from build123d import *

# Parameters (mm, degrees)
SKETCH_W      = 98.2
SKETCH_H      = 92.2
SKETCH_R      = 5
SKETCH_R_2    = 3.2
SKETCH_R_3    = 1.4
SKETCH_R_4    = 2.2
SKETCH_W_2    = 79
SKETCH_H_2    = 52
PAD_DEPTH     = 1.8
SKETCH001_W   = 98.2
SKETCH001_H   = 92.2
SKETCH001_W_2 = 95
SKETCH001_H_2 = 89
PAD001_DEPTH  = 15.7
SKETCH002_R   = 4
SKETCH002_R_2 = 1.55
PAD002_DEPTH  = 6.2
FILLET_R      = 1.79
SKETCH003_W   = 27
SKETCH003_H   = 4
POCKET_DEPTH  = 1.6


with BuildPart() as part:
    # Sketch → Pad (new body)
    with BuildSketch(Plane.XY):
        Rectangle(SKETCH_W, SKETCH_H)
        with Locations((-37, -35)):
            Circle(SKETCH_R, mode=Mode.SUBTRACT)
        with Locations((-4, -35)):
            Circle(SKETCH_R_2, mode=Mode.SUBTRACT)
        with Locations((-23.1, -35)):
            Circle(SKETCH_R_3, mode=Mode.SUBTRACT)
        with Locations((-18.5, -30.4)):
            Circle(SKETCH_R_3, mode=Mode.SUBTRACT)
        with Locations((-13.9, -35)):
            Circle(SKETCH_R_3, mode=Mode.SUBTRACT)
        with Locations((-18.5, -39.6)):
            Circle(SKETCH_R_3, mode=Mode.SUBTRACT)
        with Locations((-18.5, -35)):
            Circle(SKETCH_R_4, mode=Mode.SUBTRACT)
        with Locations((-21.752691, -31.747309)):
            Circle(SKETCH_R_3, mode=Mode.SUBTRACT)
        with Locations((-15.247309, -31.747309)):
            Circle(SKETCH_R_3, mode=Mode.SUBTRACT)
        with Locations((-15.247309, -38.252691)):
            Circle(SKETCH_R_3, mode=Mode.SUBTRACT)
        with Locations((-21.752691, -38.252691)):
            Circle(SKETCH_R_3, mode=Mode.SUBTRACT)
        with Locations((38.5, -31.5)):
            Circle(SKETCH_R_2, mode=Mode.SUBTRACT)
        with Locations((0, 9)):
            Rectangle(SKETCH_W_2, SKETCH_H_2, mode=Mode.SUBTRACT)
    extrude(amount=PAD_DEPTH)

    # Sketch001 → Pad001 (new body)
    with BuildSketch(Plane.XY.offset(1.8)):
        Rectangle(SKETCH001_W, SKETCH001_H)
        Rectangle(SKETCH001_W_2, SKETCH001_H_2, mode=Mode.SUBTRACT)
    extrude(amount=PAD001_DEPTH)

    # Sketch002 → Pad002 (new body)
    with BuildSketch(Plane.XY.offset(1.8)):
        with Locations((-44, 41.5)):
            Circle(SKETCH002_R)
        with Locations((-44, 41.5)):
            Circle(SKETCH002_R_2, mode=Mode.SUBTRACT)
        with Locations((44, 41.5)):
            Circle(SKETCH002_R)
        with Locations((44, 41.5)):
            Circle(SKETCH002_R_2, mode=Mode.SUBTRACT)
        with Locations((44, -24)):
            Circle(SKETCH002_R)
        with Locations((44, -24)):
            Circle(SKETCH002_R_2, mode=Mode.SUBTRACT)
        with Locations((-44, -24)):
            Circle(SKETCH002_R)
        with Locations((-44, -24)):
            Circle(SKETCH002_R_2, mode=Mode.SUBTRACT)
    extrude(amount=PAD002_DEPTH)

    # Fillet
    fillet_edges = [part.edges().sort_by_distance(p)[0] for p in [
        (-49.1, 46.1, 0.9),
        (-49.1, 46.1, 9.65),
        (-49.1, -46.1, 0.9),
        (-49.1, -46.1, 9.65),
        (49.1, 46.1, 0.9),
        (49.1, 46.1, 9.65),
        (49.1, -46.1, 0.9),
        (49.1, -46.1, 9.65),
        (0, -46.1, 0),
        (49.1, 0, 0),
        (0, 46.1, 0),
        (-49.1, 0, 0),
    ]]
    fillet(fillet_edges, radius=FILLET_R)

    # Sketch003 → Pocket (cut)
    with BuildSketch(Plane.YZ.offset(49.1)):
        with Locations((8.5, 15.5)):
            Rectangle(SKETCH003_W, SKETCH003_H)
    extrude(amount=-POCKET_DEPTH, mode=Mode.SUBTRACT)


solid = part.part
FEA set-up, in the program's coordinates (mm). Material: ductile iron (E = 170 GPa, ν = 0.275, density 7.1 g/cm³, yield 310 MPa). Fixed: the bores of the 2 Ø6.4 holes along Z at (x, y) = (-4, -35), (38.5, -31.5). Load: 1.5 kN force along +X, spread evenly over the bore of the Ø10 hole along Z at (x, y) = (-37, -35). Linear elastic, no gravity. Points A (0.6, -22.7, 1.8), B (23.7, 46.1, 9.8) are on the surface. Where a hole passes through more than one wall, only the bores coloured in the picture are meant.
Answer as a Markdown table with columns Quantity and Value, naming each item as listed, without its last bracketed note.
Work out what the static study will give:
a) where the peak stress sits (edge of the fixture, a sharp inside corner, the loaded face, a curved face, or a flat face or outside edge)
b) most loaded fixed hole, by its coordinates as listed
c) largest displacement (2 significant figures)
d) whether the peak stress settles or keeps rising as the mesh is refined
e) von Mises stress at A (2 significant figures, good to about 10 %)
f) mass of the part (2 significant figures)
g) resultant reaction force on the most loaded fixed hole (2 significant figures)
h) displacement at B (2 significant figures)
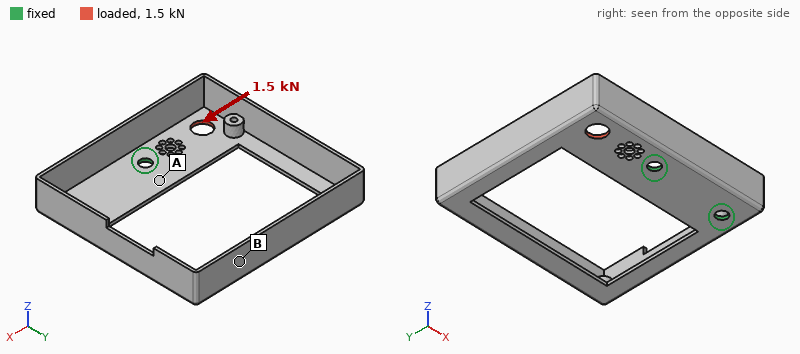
| Quantity | Value |
|---|---|
| where the peak stress sits | a sharp inside corner |
| most loaded fixed hole, by its coordinates as listed | (-4, -35) |
| largest displacement | 25 µm |
| whether the peak stress settles or keeps rising as the mesh is refined | keeps rising |
| von Mises stress at A | 12 MPa |
| mass of the part | 130 g |
| resultant reaction force on the most loaded fixed hole | 1.3 kN |
| displacement at B | 6.7 µm |
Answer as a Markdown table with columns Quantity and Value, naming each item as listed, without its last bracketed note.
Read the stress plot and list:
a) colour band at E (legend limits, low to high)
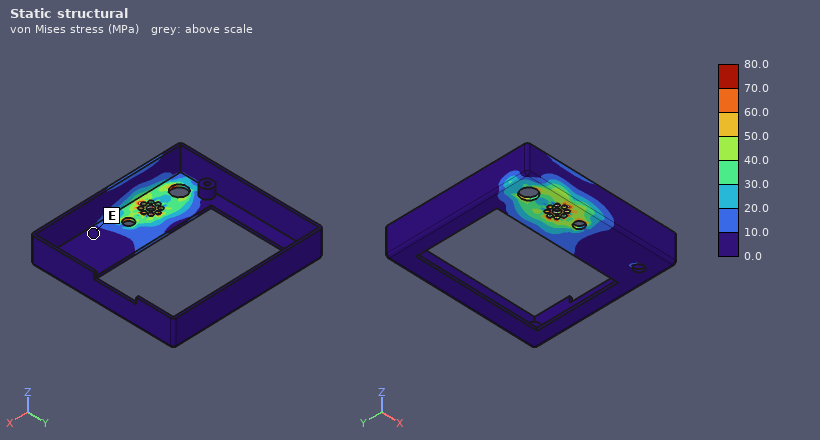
| Quantity | Value |
|---|---|
| colour band at E | 0.0 to 10.0 MPa |
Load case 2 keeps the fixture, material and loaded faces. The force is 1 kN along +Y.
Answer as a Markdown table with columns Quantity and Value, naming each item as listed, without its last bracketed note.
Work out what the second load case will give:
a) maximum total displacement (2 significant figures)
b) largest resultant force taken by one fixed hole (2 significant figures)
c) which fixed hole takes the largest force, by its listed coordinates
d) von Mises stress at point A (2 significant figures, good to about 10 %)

| Quantity | Value |
|---|---|
| maximum total displacement | 96 µm |
| largest resultant force taken by one fixed hole | 1.6 kN |
| which fixed hole takes the largest force, by its listed coordinates | (-4, -35) |
| von Mises stress at point A | 55 MPa |
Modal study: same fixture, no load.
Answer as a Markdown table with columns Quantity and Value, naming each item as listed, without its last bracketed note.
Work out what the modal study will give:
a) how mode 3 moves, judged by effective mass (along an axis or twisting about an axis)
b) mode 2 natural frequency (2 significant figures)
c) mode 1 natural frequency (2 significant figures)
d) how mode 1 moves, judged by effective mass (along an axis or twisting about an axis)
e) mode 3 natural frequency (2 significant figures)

| Quantity | Value |
|---|---|
| how mode 3 moves, judged by effective mass | along X |
| mode 2 natural frequency | 490 Hz |
| mode 1 natural frequency | 190 Hz |
| how mode 1 moves, judged by effective mass | along Z |
| mode 3 natural frequency | 1000 Hz |
